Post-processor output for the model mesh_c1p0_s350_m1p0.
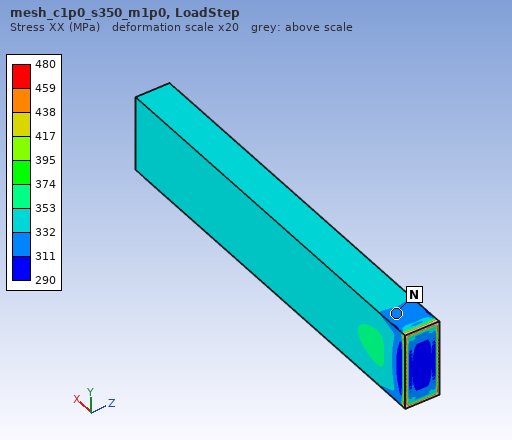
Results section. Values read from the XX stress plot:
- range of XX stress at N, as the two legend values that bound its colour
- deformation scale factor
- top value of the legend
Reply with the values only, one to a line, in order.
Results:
311 to 332 MPa
20
480 MPa
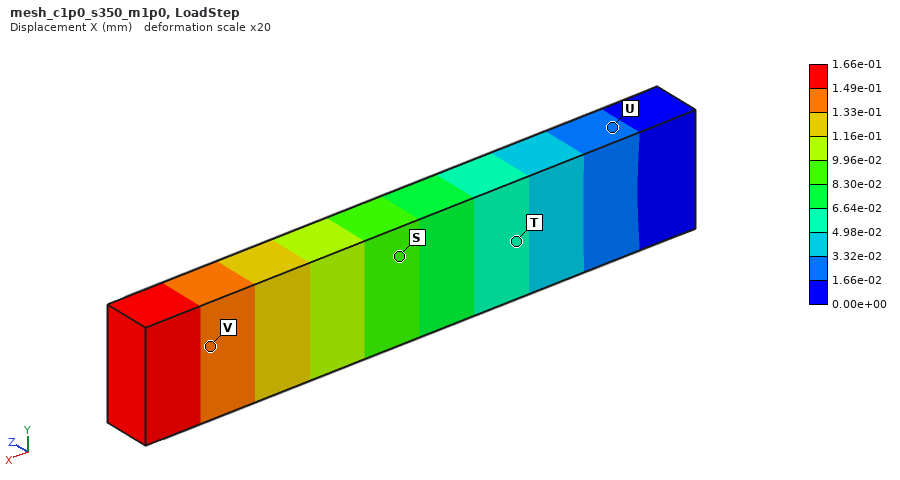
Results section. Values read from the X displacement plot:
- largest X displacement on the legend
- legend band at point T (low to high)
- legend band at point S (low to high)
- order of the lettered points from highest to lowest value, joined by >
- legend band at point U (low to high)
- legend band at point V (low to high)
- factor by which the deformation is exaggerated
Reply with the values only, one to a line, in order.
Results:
1.66e-01 mm
4.98e-02 to 6.64e-02 mm
8.30e-02 to 9.96e-02 mm
V > S > T > U
1.66e-02 to 3.32e-02 mm
1.33e-01 to 1.49e-01 mm
20
